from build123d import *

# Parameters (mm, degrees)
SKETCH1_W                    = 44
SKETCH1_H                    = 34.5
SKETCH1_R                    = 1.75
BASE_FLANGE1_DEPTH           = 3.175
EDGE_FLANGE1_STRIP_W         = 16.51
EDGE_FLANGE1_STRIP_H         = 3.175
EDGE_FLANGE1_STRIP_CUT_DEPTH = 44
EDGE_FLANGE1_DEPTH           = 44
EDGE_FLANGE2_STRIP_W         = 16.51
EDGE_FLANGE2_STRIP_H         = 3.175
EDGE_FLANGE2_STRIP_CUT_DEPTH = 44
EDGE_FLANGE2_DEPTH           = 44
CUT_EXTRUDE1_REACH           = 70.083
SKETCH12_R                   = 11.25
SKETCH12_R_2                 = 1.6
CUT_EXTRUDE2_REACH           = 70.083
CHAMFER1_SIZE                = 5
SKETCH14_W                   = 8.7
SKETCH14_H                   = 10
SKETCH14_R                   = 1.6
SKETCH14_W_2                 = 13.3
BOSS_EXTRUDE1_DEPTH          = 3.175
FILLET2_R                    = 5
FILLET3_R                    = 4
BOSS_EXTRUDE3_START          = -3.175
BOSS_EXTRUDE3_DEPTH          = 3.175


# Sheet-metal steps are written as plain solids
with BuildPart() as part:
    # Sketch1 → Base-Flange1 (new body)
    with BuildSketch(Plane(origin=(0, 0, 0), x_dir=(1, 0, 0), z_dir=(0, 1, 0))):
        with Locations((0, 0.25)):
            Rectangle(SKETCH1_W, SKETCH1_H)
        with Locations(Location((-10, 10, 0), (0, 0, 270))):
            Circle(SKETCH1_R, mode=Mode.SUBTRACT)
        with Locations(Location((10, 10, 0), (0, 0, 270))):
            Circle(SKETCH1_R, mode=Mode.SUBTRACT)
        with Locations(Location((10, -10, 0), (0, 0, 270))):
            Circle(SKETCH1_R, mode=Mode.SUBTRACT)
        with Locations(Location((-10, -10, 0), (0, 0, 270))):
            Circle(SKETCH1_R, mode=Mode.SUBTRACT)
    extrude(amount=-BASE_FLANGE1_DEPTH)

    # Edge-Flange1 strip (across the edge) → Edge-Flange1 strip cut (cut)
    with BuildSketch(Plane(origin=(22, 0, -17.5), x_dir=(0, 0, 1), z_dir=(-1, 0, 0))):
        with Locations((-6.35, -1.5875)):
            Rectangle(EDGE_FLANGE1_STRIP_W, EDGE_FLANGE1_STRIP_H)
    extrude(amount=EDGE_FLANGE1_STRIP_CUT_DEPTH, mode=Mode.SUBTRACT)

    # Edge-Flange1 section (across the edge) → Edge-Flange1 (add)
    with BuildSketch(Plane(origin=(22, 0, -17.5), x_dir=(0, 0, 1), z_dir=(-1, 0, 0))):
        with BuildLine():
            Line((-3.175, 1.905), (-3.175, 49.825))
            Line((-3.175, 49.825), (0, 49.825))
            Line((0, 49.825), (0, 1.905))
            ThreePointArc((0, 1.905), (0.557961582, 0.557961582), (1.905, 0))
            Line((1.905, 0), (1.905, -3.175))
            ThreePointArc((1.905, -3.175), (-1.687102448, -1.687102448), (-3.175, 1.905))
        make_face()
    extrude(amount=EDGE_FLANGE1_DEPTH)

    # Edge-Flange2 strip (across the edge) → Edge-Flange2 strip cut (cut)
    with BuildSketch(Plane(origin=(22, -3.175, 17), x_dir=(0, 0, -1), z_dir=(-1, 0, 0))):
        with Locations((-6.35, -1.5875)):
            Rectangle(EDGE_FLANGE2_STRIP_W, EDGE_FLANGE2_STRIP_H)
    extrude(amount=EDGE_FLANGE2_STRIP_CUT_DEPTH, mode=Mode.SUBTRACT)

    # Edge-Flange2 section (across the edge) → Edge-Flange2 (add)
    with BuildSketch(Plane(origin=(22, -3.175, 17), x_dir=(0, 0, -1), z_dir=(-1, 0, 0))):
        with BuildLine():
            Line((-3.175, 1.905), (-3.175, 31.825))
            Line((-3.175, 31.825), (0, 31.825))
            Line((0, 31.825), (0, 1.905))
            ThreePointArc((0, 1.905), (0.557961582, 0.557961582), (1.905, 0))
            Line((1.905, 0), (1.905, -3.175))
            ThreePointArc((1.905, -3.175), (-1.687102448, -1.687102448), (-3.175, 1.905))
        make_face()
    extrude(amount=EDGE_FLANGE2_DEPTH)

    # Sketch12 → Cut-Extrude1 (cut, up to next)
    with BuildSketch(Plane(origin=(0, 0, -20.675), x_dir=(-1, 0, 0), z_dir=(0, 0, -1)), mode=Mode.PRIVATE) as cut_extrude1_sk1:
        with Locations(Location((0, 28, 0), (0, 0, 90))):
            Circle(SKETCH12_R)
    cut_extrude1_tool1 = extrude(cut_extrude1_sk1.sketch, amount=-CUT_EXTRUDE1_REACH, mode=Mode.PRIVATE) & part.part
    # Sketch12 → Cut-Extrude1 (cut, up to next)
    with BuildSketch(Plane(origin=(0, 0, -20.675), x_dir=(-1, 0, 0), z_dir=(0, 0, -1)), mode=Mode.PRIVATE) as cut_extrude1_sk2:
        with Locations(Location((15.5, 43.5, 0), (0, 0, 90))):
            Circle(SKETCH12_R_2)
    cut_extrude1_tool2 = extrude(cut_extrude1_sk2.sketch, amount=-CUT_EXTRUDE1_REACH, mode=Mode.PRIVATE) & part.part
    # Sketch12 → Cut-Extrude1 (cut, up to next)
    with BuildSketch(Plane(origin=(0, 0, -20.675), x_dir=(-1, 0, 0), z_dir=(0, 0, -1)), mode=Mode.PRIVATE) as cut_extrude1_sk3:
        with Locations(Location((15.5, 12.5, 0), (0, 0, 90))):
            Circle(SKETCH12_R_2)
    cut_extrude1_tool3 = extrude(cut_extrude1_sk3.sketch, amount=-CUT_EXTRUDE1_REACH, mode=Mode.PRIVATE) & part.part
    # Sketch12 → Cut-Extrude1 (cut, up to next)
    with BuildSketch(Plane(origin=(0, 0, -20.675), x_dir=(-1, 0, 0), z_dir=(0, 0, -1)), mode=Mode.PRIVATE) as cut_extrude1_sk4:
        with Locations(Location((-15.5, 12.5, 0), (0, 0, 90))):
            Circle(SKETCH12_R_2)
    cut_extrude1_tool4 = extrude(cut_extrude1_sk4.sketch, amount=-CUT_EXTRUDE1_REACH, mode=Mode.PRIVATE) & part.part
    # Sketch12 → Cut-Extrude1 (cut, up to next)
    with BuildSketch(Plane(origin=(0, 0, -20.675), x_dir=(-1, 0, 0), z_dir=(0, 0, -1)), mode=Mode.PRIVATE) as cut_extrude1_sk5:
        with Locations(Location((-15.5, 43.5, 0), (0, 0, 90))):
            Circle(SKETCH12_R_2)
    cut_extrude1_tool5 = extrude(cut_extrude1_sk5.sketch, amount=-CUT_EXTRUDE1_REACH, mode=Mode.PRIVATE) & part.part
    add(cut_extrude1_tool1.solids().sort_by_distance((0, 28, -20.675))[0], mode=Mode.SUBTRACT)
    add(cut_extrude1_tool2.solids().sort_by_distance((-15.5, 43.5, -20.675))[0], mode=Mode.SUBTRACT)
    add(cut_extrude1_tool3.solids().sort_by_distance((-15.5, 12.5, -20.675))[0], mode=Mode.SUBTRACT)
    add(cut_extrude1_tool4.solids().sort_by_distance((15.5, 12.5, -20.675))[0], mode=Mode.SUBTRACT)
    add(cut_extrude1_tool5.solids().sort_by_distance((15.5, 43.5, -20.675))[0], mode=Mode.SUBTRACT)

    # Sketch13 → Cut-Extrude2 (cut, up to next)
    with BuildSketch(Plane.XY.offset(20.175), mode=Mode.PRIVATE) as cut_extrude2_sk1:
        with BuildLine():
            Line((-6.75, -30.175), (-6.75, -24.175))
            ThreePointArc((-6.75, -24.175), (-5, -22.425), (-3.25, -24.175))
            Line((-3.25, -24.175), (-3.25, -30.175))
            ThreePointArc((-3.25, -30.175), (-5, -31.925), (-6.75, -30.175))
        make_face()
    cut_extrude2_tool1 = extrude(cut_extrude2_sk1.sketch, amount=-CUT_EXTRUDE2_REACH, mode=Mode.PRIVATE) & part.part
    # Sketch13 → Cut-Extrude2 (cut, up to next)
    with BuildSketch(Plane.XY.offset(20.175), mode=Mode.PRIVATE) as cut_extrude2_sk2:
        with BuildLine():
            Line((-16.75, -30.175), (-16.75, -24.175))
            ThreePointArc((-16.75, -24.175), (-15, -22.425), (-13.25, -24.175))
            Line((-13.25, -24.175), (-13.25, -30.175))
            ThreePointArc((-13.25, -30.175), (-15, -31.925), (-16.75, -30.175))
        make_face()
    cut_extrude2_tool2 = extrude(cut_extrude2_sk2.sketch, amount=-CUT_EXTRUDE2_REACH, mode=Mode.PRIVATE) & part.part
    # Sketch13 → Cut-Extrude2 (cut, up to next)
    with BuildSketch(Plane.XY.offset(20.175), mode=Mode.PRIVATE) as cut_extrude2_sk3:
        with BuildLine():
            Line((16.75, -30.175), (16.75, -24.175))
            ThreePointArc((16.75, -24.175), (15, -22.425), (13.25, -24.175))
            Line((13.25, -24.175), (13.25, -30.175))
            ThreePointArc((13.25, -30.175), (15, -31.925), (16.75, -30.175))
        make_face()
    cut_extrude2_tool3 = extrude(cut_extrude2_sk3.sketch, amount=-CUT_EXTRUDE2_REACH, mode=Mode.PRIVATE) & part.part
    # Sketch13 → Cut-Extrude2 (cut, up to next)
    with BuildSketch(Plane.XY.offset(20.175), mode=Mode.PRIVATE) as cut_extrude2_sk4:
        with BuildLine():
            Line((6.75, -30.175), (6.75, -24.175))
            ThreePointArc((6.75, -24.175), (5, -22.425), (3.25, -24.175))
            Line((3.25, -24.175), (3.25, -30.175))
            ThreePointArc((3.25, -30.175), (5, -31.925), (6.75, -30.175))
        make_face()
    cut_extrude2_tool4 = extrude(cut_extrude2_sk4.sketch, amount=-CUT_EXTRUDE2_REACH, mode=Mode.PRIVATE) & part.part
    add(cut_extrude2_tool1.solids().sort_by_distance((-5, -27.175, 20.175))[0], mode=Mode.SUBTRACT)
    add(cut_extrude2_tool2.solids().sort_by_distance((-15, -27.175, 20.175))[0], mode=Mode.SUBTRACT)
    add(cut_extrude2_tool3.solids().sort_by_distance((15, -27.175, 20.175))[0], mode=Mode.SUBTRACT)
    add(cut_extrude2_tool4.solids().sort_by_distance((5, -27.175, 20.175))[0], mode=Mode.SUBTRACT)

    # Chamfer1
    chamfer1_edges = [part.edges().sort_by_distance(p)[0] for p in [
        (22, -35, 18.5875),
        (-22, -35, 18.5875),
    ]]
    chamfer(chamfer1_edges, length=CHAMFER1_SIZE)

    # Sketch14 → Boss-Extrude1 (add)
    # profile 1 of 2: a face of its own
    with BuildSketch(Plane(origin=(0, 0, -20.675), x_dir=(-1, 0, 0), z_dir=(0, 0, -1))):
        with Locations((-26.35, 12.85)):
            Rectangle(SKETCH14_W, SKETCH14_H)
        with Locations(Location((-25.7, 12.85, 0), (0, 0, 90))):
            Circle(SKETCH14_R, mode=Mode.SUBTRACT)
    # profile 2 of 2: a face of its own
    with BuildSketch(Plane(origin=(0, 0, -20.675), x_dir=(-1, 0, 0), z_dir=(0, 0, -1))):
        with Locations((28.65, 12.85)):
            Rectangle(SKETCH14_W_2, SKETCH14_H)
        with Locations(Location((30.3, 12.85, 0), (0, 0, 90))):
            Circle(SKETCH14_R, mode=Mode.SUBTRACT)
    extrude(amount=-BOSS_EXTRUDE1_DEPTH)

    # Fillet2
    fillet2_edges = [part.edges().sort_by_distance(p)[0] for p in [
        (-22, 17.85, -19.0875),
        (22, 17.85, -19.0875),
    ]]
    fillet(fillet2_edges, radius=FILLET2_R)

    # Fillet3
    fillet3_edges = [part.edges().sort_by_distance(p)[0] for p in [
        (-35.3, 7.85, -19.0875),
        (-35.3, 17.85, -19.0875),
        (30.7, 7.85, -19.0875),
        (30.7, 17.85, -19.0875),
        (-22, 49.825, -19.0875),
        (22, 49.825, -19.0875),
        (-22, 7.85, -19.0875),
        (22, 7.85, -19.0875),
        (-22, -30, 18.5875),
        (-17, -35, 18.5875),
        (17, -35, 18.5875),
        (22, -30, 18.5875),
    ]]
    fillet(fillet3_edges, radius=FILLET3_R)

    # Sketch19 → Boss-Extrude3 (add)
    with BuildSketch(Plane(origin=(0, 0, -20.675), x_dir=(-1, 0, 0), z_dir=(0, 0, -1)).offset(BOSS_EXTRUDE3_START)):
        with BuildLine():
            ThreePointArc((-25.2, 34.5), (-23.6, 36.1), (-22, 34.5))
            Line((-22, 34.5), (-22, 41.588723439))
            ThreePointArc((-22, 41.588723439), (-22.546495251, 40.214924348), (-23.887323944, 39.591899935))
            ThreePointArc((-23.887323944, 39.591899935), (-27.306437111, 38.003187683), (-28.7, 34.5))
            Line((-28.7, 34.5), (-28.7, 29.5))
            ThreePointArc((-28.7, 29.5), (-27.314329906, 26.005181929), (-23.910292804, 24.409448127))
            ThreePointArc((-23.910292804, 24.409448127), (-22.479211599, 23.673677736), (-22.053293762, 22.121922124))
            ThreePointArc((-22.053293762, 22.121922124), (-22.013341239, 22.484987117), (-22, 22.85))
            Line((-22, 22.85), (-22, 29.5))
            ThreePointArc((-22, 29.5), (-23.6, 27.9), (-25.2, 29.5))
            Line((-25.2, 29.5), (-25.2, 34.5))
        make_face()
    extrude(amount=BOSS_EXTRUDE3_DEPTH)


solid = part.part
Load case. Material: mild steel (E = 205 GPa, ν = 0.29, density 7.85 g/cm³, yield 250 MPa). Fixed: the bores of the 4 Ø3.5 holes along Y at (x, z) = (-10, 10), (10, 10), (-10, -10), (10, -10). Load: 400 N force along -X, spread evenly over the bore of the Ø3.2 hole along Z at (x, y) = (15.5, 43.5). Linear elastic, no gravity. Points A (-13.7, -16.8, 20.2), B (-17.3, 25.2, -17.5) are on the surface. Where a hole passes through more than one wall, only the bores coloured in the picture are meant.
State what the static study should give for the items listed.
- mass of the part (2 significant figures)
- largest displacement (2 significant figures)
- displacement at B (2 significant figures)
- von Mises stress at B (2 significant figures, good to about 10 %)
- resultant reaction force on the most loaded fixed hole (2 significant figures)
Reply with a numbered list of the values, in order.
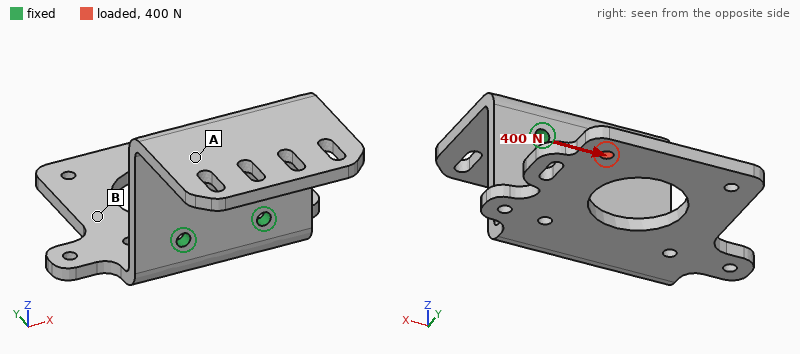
1. 120 g
2. 72 µm
3. 42 µm
4. 23 MPa
5. 830 N
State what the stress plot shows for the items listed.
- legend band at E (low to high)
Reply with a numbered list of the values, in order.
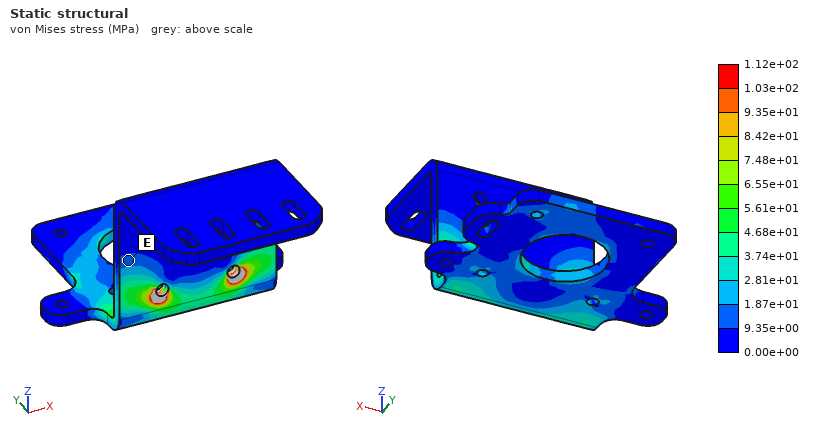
1. 9.35e+00 to 1.87e+01 MPa
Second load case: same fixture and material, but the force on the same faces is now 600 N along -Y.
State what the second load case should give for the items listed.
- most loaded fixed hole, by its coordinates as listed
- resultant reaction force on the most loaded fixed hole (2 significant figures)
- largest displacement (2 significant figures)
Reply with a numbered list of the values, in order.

1. (10, -10)
2. 750 N
3. 79 µm
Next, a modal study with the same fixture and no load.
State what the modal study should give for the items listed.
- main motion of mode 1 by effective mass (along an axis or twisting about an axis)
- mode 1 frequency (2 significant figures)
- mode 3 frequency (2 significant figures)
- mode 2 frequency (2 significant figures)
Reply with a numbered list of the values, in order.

1. along Z
2. 820 Hz
3. 2000 Hz
4. 1900 Hz
